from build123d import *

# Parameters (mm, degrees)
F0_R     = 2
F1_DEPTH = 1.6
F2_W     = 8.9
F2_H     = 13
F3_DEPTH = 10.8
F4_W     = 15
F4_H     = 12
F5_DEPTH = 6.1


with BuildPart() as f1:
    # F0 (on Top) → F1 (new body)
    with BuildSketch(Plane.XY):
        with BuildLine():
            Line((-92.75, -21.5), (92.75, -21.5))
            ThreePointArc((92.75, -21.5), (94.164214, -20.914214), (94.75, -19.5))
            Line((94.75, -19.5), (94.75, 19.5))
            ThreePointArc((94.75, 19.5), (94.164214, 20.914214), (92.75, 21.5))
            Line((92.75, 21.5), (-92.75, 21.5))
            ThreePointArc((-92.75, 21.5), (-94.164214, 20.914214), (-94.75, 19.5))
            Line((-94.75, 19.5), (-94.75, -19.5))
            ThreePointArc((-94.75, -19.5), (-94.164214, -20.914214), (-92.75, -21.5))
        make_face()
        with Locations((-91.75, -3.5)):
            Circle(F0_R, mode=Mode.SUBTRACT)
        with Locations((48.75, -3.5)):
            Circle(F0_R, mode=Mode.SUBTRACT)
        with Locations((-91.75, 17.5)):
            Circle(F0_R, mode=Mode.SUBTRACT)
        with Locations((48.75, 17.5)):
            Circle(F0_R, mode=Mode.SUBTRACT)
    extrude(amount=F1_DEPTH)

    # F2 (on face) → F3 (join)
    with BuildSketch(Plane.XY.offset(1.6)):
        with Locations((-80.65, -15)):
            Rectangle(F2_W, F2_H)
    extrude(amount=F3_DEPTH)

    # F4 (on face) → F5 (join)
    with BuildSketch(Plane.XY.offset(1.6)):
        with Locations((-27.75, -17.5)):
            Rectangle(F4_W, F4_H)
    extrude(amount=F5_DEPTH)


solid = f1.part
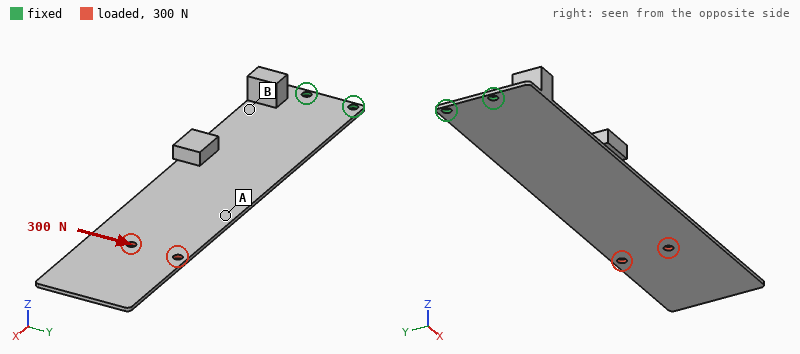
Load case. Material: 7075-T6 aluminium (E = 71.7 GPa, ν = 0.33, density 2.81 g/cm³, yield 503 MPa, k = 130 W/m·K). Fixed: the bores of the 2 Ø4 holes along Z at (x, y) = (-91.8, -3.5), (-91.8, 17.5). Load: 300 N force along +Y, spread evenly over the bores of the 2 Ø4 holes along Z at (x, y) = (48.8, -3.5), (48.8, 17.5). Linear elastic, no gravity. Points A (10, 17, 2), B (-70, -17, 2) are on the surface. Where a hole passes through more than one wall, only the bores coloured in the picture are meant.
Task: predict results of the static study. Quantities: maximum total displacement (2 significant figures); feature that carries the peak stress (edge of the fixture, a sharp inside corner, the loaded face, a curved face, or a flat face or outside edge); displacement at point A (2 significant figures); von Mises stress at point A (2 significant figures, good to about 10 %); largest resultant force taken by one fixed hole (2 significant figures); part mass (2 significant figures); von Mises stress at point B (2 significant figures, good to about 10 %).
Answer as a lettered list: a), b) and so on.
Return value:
a) 0.82 mm
b) edge of the fixture
c) 0.37 mm
d) 19 MPa
e) 1.9 kN
f) 43 g
g) 51 MPa
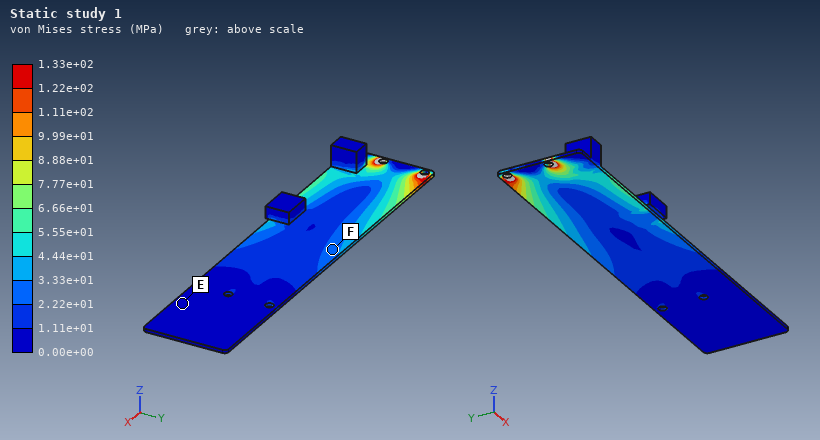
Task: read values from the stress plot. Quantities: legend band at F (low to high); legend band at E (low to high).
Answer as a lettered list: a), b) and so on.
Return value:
a) 2.22e+01 to 3.33e+01 MPa
b) 0.00e+00 to 1.11e+01 MPa
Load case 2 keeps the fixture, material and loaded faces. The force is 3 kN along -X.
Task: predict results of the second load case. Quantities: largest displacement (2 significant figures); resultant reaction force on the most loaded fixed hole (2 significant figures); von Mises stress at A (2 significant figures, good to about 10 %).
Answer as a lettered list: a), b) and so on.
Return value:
a) 0.45 mm
b) 1.5 kN
c) 77 MPa
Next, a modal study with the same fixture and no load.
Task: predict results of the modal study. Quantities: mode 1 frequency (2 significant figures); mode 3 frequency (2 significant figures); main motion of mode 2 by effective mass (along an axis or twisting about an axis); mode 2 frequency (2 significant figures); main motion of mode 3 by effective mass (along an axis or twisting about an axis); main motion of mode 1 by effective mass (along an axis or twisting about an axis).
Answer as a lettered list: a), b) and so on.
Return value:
a) 40 Hz
b) 320 Hz
c) along Z
d) 230 Hz
e) twisting about X
f) along Z
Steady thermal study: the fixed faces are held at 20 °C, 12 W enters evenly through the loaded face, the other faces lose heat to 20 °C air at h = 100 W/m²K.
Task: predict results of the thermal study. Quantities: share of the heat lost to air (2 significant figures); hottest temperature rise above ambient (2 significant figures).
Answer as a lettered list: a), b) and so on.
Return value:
a) 99 %
b) 32 K
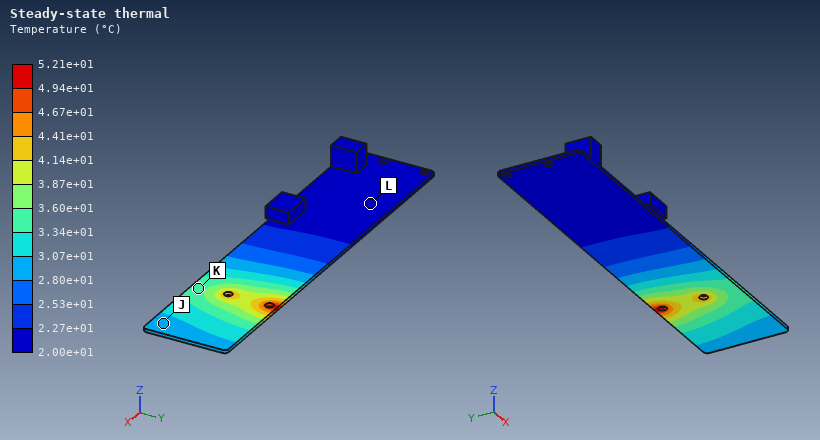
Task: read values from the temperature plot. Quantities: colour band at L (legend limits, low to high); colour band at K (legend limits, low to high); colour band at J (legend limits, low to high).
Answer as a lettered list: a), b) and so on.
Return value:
a) 2.00e+01 to 2.27e+01 °C
b) 3.34e+01 to 3.60e+01 °C
c) 2.80e+01 to 3.07e+01 °C
